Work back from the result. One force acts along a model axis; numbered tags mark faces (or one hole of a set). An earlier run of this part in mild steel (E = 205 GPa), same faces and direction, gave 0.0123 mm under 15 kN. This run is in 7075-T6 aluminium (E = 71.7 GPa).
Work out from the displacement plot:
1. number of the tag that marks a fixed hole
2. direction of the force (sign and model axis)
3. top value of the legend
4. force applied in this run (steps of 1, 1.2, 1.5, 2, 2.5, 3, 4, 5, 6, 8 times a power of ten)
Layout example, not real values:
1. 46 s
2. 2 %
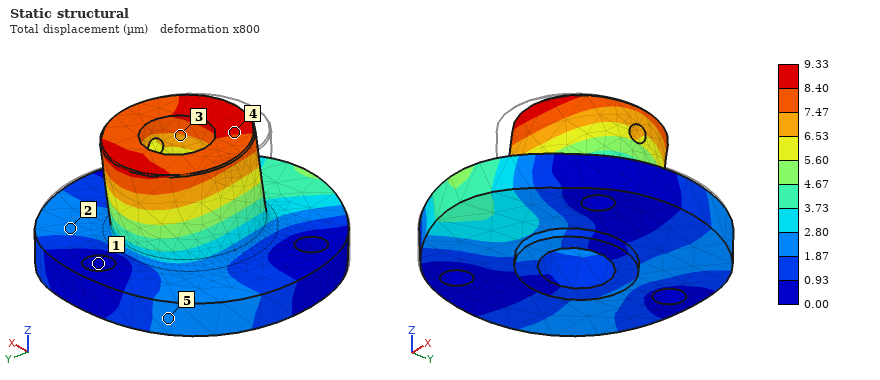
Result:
1. 1
2. +Y
3. 9.33 µm
4. 4 kN
